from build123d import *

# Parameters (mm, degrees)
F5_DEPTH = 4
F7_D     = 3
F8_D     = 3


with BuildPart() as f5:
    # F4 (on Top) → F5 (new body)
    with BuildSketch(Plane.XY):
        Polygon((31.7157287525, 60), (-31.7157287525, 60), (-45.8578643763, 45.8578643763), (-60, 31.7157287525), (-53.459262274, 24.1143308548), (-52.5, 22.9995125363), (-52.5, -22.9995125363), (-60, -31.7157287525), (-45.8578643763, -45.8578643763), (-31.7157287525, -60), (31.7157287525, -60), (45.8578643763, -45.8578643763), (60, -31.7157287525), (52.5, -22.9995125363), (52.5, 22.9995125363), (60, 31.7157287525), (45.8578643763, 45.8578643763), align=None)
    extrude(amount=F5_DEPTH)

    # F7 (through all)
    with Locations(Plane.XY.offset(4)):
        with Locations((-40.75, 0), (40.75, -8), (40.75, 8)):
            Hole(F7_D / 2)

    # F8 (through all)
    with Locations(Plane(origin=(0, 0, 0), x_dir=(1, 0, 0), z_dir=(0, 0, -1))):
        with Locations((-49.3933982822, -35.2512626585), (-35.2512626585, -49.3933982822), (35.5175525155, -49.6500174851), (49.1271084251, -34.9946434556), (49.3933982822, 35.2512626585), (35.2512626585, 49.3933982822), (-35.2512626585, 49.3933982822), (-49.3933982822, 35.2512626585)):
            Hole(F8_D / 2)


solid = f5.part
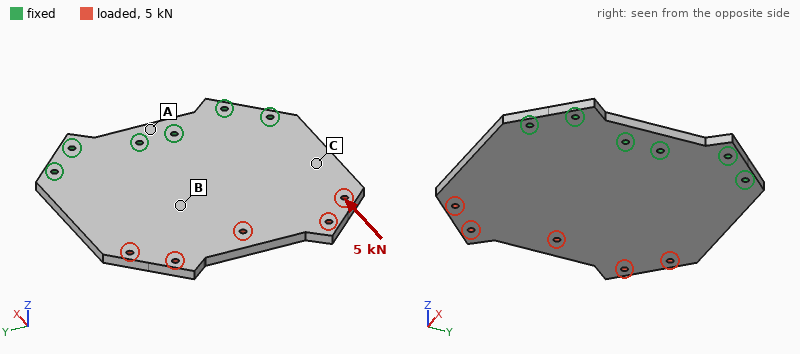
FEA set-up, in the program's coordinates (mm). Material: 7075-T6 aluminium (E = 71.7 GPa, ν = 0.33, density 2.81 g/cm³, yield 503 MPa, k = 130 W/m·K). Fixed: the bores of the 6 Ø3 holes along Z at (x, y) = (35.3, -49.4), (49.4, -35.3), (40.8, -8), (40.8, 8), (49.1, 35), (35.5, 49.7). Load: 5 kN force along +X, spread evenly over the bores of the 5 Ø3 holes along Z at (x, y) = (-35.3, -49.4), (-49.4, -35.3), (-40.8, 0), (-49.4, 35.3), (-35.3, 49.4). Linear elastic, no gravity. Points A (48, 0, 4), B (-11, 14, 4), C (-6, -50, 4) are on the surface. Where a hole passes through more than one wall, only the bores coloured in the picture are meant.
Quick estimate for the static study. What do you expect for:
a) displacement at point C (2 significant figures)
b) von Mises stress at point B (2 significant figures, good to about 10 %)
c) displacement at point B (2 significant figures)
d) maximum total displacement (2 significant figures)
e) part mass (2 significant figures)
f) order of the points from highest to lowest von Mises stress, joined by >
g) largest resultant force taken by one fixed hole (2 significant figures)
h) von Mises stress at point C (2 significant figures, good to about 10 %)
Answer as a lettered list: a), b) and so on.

a) 8.6 µm
b) 8.4 MPa
c) 7.6 µm
d) 17 µm
e) 130 g
f) C > B > A
g) 1.1 kN
h) 12 MPa
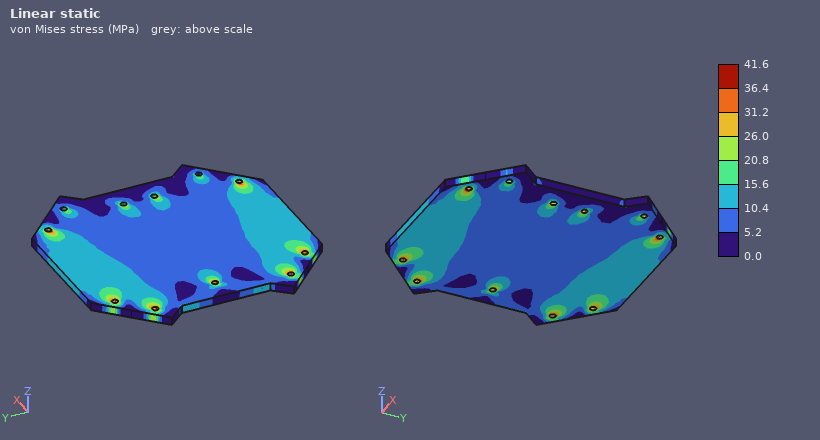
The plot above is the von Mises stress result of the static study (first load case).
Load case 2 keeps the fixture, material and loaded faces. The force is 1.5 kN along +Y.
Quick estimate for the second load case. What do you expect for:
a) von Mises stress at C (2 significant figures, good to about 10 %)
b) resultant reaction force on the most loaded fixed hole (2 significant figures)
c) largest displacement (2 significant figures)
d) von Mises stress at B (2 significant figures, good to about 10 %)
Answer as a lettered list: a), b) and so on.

a) 5.3 MPa
b) 1.0 kN
c) 23 µm
d) 7.7 MPa
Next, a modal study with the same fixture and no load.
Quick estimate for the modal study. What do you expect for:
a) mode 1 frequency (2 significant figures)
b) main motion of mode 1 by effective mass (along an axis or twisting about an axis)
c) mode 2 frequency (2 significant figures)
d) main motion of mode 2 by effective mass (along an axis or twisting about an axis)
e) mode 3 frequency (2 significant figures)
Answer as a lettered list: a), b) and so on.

a) 400 Hz
b) along Z
c) 910 Hz
d) twisting about X
e) 2100 Hz
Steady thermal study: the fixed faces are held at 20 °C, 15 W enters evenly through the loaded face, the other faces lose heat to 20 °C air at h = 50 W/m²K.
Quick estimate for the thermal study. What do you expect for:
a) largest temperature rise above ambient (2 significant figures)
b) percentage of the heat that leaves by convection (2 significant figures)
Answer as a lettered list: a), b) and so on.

a) 15 K
b) 50 %
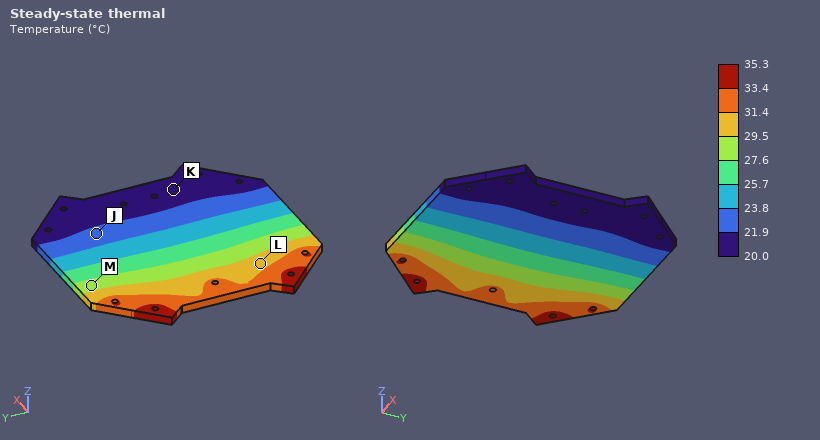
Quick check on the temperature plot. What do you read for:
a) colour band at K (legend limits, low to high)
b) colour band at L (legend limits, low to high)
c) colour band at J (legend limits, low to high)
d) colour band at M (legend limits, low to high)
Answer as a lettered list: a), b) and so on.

a) 20.0 to 21.9 °C
b) 29.5 to 31.4 °C
c) 21.9 to 23.8 °C
d) 27.6 to 29.5 °C
